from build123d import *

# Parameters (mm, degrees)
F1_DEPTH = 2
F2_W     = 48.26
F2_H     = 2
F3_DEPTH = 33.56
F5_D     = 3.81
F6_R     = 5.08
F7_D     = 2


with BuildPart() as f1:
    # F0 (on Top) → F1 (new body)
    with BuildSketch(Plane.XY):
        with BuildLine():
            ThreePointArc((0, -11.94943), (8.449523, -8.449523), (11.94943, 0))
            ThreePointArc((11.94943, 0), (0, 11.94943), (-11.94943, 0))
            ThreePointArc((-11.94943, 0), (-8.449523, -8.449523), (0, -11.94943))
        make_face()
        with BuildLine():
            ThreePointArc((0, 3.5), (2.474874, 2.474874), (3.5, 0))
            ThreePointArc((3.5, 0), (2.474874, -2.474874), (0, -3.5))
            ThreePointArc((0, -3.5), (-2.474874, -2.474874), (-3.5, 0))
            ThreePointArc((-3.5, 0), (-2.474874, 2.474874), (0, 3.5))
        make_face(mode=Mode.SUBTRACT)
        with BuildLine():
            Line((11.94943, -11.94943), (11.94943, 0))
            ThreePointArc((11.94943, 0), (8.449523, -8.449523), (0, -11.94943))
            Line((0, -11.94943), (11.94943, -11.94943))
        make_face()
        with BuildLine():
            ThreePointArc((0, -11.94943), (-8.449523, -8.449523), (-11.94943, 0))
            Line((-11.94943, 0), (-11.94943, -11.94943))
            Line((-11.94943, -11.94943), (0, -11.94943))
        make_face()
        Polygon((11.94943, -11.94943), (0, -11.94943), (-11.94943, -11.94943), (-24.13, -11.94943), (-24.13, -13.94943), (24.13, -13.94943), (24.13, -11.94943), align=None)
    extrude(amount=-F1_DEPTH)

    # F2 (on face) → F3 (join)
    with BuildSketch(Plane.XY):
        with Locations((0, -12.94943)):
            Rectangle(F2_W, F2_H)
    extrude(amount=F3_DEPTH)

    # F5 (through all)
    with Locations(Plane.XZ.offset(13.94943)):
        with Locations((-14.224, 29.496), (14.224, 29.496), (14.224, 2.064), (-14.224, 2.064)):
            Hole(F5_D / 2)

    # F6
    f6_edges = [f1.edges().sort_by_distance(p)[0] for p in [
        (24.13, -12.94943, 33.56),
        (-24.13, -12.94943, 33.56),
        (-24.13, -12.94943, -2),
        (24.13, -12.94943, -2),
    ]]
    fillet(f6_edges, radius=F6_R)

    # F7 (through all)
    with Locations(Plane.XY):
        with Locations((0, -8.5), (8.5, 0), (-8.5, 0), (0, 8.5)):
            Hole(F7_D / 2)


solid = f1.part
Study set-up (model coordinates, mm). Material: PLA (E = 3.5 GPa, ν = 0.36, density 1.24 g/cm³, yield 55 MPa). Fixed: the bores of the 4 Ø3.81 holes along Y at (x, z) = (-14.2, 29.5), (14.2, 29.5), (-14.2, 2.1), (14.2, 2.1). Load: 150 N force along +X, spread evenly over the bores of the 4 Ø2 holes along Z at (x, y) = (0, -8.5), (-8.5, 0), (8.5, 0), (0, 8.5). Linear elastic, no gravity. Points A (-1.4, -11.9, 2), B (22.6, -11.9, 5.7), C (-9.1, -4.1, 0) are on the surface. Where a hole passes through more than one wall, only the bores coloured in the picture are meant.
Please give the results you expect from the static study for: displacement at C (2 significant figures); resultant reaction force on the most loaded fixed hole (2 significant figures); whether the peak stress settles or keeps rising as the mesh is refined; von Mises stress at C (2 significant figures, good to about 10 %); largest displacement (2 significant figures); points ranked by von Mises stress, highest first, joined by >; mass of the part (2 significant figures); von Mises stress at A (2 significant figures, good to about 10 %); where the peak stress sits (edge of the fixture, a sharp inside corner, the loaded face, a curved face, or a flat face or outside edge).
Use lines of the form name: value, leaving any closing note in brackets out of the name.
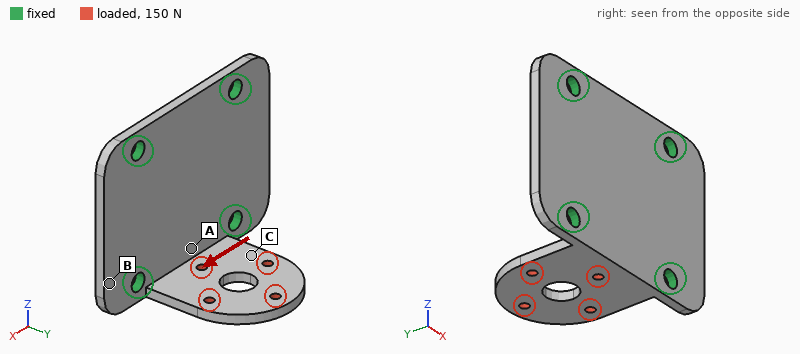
displacement at C: 0.098 mm
resultant reaction force on the most loaded fixed hole: 110 N
whether the peak stress settles or keeps rising as the mesh is refined: keeps rising
von Mises stress at C: 7.1 MPa
largest displacement: 0.19 mm
points ranked by von Mises stress, highest first, joined by >: C > A > B
mass of the part: 5.2 g
von Mises stress at A: 4.6 MPa
where the peak stress sits: edge of the fixture
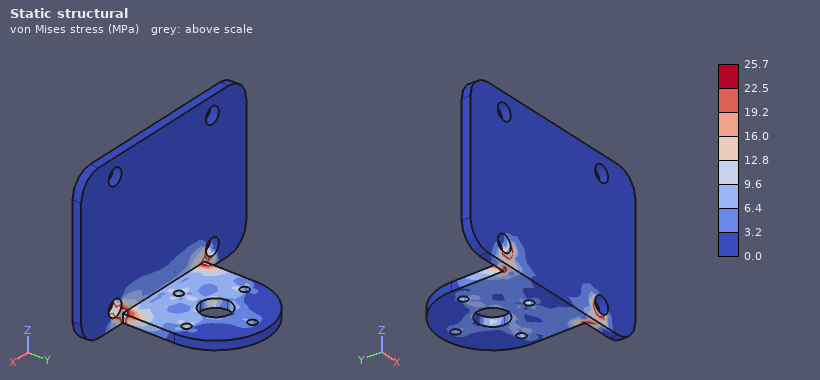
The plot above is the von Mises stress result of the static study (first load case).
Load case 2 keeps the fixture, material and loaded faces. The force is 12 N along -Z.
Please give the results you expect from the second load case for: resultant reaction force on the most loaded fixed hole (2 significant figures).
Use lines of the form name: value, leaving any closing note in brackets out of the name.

resultant reaction force on the most loaded fixed hole: 4.9 N
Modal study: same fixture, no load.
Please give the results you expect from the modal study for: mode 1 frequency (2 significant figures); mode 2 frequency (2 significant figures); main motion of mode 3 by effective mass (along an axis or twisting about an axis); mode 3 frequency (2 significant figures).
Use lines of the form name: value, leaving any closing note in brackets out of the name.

mode 1 frequency: 890 Hz
mode 2 frequency: 2600 Hz
main motion of mode 3 by effective mass: along Y
mode 3 frequency: 3700 Hz
